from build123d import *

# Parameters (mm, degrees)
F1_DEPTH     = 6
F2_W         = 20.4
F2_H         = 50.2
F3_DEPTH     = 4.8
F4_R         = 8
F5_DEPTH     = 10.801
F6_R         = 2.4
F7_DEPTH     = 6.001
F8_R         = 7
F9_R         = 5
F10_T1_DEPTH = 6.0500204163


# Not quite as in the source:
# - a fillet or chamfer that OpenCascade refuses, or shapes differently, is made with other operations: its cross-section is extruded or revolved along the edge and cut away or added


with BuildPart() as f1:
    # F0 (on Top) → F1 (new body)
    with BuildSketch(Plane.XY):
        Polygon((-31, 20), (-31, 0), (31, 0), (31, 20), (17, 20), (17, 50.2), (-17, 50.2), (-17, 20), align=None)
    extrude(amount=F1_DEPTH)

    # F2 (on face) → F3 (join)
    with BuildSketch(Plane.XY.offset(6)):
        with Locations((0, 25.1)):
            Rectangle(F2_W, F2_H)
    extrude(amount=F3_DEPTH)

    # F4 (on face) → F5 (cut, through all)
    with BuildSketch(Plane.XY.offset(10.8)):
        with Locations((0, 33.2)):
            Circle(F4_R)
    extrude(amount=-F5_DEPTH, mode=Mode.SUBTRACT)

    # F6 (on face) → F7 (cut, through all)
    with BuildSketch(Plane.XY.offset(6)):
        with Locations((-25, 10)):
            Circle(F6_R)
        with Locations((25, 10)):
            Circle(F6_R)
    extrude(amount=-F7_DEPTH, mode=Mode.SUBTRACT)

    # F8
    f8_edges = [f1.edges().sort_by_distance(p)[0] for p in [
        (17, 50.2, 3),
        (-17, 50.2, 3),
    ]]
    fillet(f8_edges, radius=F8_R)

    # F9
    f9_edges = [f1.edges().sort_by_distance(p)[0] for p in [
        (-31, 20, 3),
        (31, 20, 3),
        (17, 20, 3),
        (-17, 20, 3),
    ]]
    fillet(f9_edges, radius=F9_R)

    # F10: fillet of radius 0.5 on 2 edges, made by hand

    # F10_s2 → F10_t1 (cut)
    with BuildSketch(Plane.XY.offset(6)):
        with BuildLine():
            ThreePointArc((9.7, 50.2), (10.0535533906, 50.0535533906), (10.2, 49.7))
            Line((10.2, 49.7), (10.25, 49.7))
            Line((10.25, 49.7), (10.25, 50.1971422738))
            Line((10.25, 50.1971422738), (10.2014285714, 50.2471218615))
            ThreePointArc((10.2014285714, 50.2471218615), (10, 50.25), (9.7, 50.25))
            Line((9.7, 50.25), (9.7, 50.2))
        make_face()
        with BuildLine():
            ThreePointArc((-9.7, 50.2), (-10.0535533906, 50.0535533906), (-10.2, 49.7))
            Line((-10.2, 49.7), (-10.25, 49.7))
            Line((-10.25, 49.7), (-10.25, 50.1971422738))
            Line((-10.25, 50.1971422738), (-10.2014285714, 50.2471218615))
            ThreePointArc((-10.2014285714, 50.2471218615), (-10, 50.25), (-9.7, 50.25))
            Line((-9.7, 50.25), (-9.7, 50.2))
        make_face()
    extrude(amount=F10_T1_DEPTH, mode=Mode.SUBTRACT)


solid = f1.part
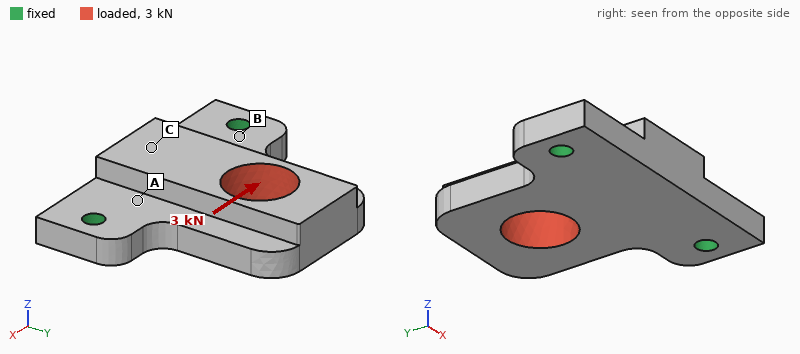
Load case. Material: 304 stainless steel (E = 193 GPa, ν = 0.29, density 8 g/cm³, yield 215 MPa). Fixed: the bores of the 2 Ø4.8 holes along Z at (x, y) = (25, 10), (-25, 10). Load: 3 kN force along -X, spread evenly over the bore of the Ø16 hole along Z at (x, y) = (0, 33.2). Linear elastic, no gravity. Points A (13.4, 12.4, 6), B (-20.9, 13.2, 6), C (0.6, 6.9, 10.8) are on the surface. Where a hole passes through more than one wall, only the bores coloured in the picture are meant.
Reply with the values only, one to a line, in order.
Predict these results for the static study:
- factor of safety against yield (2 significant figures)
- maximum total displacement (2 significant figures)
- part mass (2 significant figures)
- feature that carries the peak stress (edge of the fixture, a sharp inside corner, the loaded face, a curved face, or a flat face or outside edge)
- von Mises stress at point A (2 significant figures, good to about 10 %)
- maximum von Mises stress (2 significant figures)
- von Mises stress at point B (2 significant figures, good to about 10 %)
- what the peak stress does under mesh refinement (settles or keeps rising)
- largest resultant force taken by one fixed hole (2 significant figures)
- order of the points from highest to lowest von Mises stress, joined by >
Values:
2.3
14 µm
130 g
a curved face
18 MPa
94 MPa
35 MPa
settles
2.1 kN
B > A > C
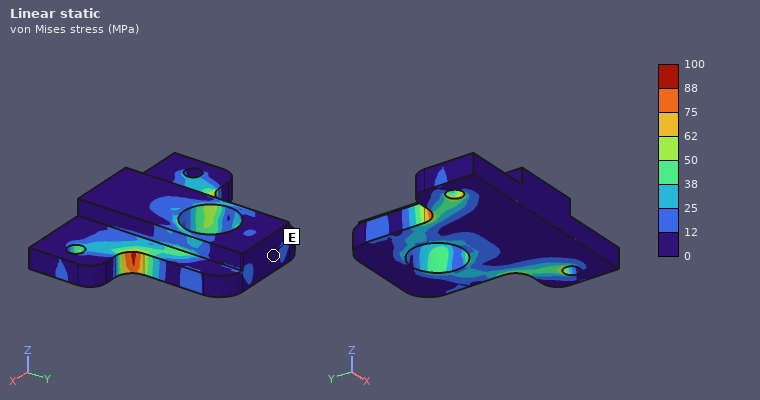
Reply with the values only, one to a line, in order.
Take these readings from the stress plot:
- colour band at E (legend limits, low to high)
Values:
0 to 12 MPa
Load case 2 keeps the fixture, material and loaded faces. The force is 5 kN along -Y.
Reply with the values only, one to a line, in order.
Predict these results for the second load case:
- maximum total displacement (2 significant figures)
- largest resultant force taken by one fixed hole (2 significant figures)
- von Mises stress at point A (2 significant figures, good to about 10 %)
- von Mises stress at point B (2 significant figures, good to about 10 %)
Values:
50 µm
2.6 kN
55 MPa
110 MPa
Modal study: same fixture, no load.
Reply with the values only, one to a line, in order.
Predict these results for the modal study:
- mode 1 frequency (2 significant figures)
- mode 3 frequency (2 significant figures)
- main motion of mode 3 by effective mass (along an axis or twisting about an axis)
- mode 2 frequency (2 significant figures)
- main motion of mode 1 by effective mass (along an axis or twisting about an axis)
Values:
2600 Hz
10 kHz
along X
9300 Hz
along Z
